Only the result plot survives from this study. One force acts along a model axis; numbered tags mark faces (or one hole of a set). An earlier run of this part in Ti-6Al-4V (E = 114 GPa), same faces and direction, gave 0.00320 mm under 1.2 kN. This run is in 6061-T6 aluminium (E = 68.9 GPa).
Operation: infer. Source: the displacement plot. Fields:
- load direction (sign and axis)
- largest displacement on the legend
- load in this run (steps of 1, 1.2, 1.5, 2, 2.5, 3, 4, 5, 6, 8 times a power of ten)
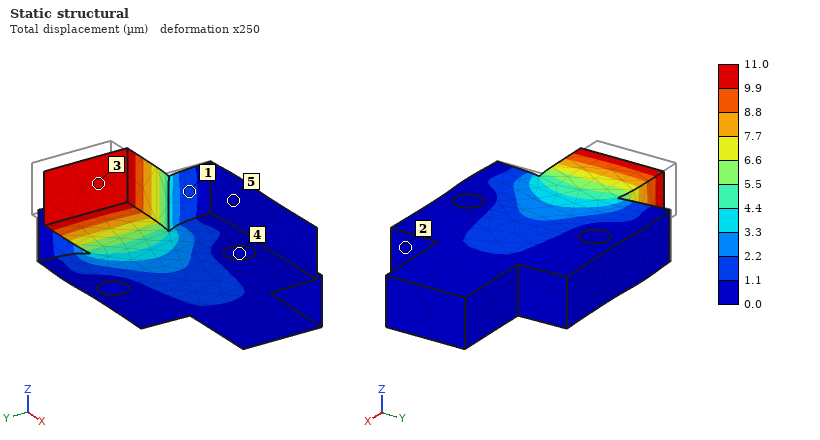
+X
11.0 µm
2.5 kN
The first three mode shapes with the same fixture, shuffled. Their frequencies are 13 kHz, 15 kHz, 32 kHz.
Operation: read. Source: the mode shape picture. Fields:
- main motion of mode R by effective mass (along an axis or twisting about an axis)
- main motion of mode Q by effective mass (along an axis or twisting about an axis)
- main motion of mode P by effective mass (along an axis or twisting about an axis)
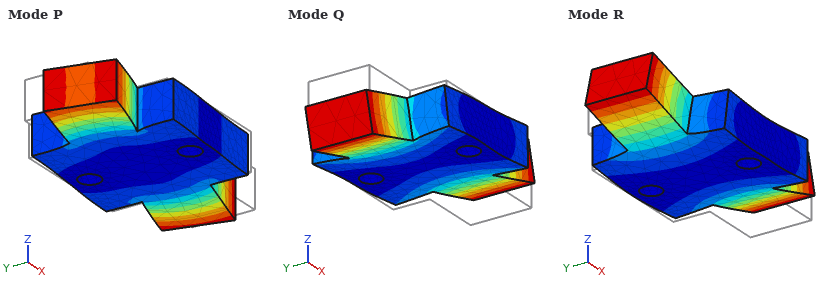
along Z
twisting about Y
twisting about Z
